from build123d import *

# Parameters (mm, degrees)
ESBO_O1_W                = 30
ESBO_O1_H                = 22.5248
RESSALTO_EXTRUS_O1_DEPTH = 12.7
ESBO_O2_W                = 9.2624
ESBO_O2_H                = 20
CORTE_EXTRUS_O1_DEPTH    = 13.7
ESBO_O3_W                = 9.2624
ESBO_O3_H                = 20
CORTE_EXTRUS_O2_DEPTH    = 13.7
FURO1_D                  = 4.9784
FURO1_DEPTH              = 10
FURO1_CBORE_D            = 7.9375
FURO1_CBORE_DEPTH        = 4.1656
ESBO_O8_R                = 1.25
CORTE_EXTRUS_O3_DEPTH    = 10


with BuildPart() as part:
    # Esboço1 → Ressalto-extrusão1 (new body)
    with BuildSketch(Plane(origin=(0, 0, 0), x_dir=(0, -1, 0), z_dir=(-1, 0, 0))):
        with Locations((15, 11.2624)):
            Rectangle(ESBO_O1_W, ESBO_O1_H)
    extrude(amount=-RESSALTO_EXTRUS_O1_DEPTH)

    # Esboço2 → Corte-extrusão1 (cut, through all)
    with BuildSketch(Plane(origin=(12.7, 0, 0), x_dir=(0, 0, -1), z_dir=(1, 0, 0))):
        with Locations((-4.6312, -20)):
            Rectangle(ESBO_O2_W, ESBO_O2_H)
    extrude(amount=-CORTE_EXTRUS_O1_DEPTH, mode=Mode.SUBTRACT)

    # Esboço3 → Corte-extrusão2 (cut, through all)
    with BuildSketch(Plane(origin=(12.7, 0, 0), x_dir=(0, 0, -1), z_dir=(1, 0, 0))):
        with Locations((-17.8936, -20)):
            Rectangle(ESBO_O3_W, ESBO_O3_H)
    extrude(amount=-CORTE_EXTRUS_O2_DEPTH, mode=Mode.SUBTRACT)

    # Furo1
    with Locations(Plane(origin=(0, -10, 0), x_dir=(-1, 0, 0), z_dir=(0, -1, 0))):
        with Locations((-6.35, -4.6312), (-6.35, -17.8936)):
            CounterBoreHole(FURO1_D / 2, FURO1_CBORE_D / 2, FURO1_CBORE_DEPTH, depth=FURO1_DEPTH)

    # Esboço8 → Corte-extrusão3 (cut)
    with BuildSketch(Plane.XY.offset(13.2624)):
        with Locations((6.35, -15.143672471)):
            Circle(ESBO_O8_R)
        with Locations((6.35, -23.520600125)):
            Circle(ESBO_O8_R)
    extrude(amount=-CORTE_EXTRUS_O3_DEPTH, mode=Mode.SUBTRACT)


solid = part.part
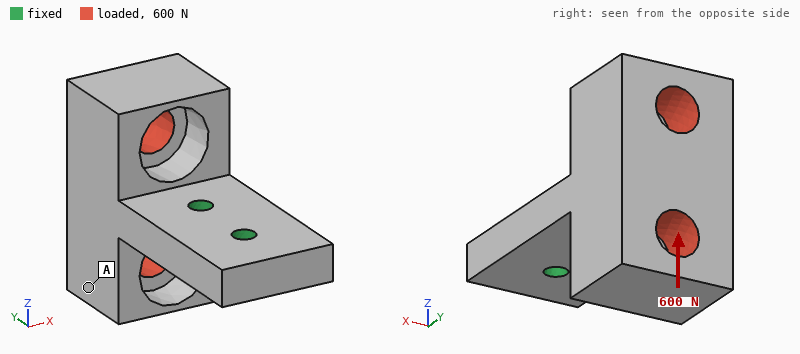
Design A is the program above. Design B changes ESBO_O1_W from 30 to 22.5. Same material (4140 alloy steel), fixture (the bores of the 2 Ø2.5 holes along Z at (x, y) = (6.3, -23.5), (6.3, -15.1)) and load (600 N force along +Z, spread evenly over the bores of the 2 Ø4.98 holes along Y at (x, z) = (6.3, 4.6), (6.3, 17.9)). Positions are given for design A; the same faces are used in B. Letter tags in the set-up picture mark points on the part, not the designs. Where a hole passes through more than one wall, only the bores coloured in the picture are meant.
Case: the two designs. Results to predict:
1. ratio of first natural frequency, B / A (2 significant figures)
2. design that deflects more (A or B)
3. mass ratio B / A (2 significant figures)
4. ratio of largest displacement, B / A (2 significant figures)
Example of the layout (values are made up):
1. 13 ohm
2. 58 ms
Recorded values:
1. 1.5
2. A
3. 0.65
4. 0.69
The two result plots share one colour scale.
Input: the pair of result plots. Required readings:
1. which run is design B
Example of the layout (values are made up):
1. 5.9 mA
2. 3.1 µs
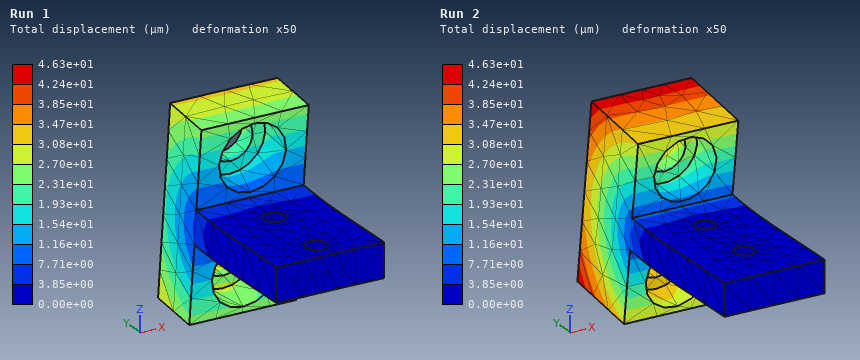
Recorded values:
1. Run 1
